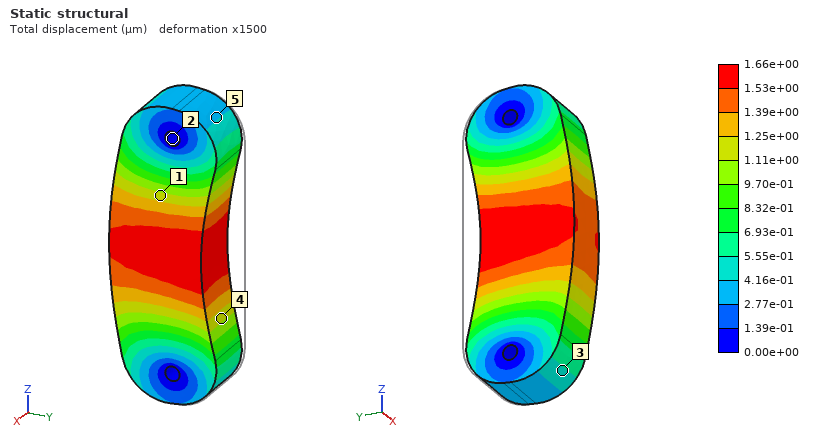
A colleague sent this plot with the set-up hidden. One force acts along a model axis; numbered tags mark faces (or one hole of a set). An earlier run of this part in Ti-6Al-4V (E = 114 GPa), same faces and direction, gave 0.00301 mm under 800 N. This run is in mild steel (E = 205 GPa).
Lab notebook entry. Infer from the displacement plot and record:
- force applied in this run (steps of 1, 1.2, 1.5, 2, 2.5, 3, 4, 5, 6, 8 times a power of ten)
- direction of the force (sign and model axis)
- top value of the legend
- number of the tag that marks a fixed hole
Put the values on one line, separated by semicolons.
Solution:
800 N; -Y; 1.66e+00 µm; 2
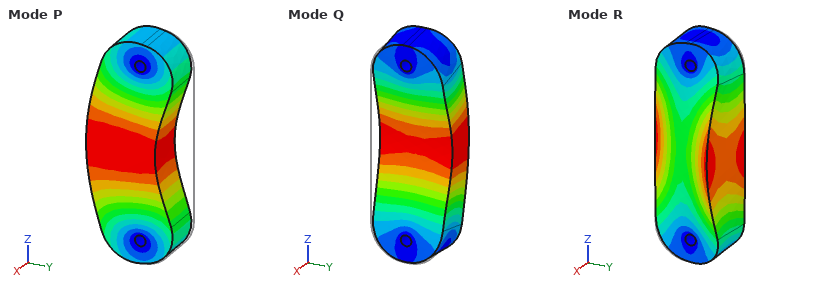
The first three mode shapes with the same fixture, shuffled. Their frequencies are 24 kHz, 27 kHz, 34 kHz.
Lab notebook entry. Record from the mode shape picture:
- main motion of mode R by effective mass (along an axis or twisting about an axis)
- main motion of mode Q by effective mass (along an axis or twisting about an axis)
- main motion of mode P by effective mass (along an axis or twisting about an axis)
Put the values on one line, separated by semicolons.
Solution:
twisting about Z; along X; along Y
